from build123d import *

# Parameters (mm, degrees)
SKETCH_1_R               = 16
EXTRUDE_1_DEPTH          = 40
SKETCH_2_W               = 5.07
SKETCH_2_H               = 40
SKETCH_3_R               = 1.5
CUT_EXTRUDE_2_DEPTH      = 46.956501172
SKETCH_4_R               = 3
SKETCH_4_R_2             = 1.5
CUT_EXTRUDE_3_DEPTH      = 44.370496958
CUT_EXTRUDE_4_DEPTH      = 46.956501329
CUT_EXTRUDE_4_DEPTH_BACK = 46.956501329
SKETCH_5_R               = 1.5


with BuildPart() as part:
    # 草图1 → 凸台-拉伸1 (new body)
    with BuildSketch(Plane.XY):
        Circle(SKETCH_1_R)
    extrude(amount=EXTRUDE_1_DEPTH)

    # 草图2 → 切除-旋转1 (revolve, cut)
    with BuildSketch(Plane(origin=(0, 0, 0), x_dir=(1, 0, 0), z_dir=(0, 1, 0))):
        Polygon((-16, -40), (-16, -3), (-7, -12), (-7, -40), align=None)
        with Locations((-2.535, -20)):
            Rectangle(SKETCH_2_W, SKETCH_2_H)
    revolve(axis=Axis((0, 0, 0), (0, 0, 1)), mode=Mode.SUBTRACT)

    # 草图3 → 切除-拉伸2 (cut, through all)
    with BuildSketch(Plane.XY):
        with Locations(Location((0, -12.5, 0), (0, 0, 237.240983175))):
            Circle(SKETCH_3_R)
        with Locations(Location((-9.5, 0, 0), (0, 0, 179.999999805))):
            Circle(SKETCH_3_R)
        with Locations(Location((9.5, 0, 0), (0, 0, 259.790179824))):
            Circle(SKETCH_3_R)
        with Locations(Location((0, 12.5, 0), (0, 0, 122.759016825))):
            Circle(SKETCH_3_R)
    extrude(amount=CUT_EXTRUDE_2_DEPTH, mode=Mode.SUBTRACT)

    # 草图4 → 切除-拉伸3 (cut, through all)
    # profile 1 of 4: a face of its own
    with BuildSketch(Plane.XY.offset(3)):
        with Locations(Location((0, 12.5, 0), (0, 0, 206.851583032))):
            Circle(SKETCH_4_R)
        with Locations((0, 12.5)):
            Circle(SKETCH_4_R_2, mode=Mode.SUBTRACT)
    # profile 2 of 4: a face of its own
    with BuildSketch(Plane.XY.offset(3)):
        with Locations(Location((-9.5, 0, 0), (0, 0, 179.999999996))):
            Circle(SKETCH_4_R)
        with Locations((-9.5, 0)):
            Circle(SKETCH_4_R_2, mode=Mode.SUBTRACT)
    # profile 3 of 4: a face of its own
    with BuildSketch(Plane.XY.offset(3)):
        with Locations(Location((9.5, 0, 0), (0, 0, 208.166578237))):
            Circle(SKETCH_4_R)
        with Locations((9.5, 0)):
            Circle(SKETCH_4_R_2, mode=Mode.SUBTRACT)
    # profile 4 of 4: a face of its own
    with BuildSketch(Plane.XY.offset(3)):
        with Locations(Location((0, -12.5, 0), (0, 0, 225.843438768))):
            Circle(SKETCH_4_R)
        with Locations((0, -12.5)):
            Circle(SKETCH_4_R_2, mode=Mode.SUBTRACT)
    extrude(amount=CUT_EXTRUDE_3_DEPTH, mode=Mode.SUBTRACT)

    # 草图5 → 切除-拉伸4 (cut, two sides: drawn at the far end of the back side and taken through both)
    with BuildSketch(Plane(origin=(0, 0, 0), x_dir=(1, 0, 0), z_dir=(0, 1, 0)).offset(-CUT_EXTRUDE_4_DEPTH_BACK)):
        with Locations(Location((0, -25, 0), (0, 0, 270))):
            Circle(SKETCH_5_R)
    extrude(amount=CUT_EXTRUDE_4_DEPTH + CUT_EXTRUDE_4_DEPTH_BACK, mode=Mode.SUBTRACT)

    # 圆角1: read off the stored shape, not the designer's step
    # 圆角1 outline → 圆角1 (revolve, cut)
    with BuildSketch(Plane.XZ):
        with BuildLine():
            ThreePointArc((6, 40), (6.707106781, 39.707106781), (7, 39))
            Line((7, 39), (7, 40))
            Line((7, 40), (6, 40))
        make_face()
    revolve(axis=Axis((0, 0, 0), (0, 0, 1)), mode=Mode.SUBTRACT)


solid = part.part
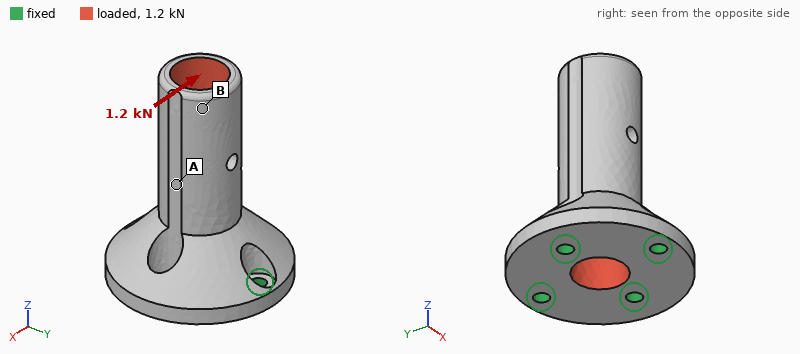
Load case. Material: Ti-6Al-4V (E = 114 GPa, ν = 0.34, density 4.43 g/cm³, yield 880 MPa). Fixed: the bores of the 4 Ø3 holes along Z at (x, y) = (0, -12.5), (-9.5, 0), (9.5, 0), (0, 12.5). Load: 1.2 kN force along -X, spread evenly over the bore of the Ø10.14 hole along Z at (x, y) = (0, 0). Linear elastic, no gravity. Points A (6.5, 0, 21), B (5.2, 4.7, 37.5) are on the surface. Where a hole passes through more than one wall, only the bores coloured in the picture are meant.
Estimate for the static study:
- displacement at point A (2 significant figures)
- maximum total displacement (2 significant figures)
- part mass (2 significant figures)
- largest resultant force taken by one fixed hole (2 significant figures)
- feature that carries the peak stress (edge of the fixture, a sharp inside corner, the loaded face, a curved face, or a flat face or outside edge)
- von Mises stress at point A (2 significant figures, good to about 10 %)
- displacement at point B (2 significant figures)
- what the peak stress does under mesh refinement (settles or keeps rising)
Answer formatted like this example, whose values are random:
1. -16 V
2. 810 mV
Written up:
1. 18 µm
2. 45 µm
3. 30 g
4. 1.1 kN
5. edge of the fixture
6. 32 MPa
7. 41 µm
8. keeps rising
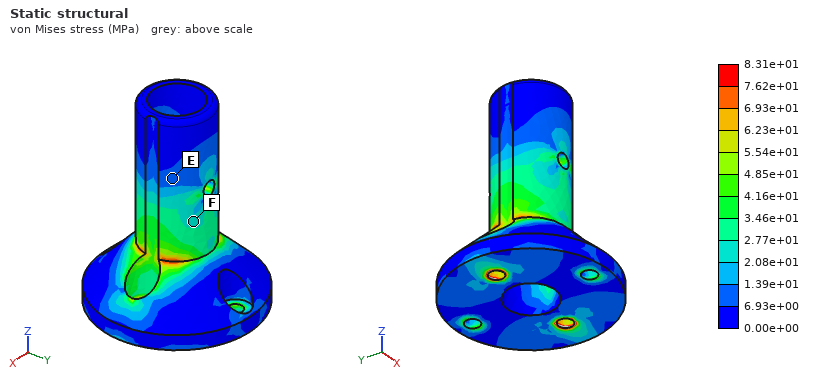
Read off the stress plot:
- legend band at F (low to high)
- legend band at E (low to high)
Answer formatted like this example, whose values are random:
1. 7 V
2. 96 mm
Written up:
1. 2.08e+01 to 2.77e+01 MPa
2. 6.93e+00 to 1.39e+01 MPa
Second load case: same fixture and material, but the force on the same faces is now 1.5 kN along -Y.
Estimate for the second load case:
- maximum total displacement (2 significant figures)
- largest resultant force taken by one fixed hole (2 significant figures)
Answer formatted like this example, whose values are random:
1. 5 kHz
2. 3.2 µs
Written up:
1. 50 µm
2. 1.2 kN
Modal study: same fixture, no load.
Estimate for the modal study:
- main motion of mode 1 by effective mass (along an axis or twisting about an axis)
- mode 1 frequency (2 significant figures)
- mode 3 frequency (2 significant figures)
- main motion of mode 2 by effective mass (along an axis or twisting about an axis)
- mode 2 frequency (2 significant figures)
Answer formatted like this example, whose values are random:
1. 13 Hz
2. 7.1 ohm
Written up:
1. along X
2. 8900 Hz
3. 24 kHz
4. along Y
5. 9400 Hz
